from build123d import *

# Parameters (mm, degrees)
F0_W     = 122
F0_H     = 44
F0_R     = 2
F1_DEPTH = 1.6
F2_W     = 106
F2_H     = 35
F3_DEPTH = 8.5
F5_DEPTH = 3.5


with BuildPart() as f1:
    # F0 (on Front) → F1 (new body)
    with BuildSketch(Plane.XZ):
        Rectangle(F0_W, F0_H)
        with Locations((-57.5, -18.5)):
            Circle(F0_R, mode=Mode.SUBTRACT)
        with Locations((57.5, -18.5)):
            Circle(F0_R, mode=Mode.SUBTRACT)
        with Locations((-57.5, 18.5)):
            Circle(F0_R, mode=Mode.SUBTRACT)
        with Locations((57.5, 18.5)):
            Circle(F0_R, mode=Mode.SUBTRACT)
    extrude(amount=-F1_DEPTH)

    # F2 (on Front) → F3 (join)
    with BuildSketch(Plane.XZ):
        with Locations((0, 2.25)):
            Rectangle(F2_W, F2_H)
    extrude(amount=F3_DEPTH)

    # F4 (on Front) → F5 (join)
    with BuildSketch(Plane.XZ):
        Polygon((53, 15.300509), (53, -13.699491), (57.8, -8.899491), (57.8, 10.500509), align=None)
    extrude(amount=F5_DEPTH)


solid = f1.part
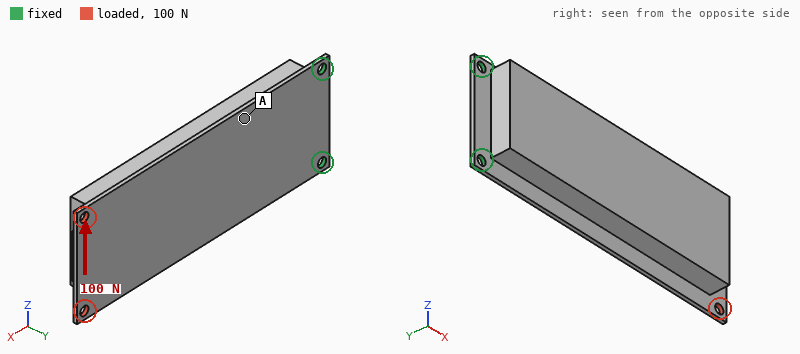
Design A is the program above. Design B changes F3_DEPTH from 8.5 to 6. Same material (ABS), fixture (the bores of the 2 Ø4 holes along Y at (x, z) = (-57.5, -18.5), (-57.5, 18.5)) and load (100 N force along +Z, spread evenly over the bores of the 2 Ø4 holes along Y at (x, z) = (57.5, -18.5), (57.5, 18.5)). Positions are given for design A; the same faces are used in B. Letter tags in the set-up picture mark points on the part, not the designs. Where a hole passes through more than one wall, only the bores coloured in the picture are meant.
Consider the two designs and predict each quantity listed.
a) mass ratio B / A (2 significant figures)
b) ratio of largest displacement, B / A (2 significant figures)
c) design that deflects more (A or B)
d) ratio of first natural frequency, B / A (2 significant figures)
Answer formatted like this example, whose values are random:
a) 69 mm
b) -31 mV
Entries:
a) 0.77
b) 1.2
c) B
d) 1.1
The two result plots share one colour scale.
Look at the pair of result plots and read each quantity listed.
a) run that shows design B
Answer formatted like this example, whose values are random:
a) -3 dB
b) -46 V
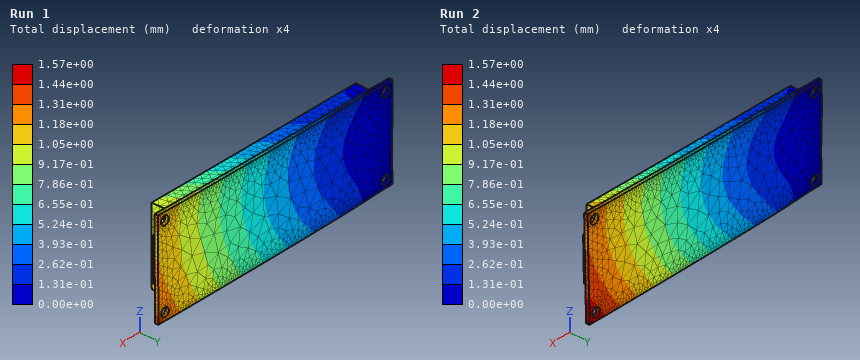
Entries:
a) Run 2
